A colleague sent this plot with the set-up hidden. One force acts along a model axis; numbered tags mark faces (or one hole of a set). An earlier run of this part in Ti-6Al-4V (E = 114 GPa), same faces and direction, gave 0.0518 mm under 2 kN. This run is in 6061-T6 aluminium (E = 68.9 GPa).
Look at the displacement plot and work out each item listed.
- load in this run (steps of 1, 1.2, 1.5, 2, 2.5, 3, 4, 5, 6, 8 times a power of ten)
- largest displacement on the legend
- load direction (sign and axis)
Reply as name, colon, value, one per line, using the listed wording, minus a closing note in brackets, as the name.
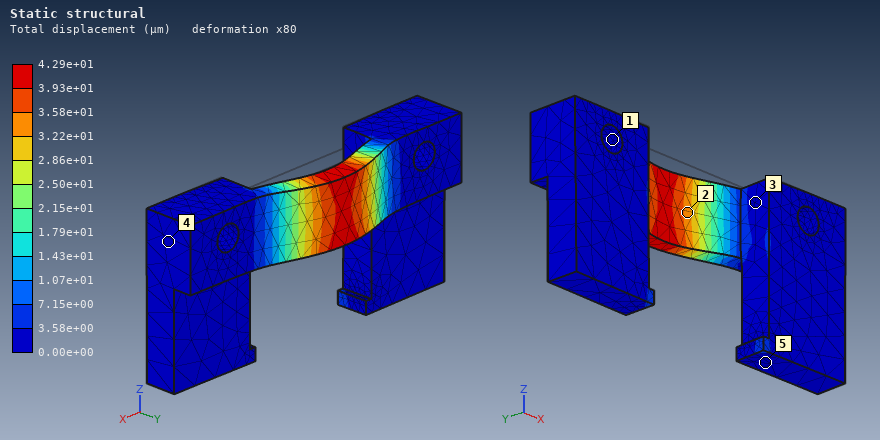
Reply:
load in this run: 1 kN
largest displacement on the legend: 4.29e+01 µm
load direction: +Y
